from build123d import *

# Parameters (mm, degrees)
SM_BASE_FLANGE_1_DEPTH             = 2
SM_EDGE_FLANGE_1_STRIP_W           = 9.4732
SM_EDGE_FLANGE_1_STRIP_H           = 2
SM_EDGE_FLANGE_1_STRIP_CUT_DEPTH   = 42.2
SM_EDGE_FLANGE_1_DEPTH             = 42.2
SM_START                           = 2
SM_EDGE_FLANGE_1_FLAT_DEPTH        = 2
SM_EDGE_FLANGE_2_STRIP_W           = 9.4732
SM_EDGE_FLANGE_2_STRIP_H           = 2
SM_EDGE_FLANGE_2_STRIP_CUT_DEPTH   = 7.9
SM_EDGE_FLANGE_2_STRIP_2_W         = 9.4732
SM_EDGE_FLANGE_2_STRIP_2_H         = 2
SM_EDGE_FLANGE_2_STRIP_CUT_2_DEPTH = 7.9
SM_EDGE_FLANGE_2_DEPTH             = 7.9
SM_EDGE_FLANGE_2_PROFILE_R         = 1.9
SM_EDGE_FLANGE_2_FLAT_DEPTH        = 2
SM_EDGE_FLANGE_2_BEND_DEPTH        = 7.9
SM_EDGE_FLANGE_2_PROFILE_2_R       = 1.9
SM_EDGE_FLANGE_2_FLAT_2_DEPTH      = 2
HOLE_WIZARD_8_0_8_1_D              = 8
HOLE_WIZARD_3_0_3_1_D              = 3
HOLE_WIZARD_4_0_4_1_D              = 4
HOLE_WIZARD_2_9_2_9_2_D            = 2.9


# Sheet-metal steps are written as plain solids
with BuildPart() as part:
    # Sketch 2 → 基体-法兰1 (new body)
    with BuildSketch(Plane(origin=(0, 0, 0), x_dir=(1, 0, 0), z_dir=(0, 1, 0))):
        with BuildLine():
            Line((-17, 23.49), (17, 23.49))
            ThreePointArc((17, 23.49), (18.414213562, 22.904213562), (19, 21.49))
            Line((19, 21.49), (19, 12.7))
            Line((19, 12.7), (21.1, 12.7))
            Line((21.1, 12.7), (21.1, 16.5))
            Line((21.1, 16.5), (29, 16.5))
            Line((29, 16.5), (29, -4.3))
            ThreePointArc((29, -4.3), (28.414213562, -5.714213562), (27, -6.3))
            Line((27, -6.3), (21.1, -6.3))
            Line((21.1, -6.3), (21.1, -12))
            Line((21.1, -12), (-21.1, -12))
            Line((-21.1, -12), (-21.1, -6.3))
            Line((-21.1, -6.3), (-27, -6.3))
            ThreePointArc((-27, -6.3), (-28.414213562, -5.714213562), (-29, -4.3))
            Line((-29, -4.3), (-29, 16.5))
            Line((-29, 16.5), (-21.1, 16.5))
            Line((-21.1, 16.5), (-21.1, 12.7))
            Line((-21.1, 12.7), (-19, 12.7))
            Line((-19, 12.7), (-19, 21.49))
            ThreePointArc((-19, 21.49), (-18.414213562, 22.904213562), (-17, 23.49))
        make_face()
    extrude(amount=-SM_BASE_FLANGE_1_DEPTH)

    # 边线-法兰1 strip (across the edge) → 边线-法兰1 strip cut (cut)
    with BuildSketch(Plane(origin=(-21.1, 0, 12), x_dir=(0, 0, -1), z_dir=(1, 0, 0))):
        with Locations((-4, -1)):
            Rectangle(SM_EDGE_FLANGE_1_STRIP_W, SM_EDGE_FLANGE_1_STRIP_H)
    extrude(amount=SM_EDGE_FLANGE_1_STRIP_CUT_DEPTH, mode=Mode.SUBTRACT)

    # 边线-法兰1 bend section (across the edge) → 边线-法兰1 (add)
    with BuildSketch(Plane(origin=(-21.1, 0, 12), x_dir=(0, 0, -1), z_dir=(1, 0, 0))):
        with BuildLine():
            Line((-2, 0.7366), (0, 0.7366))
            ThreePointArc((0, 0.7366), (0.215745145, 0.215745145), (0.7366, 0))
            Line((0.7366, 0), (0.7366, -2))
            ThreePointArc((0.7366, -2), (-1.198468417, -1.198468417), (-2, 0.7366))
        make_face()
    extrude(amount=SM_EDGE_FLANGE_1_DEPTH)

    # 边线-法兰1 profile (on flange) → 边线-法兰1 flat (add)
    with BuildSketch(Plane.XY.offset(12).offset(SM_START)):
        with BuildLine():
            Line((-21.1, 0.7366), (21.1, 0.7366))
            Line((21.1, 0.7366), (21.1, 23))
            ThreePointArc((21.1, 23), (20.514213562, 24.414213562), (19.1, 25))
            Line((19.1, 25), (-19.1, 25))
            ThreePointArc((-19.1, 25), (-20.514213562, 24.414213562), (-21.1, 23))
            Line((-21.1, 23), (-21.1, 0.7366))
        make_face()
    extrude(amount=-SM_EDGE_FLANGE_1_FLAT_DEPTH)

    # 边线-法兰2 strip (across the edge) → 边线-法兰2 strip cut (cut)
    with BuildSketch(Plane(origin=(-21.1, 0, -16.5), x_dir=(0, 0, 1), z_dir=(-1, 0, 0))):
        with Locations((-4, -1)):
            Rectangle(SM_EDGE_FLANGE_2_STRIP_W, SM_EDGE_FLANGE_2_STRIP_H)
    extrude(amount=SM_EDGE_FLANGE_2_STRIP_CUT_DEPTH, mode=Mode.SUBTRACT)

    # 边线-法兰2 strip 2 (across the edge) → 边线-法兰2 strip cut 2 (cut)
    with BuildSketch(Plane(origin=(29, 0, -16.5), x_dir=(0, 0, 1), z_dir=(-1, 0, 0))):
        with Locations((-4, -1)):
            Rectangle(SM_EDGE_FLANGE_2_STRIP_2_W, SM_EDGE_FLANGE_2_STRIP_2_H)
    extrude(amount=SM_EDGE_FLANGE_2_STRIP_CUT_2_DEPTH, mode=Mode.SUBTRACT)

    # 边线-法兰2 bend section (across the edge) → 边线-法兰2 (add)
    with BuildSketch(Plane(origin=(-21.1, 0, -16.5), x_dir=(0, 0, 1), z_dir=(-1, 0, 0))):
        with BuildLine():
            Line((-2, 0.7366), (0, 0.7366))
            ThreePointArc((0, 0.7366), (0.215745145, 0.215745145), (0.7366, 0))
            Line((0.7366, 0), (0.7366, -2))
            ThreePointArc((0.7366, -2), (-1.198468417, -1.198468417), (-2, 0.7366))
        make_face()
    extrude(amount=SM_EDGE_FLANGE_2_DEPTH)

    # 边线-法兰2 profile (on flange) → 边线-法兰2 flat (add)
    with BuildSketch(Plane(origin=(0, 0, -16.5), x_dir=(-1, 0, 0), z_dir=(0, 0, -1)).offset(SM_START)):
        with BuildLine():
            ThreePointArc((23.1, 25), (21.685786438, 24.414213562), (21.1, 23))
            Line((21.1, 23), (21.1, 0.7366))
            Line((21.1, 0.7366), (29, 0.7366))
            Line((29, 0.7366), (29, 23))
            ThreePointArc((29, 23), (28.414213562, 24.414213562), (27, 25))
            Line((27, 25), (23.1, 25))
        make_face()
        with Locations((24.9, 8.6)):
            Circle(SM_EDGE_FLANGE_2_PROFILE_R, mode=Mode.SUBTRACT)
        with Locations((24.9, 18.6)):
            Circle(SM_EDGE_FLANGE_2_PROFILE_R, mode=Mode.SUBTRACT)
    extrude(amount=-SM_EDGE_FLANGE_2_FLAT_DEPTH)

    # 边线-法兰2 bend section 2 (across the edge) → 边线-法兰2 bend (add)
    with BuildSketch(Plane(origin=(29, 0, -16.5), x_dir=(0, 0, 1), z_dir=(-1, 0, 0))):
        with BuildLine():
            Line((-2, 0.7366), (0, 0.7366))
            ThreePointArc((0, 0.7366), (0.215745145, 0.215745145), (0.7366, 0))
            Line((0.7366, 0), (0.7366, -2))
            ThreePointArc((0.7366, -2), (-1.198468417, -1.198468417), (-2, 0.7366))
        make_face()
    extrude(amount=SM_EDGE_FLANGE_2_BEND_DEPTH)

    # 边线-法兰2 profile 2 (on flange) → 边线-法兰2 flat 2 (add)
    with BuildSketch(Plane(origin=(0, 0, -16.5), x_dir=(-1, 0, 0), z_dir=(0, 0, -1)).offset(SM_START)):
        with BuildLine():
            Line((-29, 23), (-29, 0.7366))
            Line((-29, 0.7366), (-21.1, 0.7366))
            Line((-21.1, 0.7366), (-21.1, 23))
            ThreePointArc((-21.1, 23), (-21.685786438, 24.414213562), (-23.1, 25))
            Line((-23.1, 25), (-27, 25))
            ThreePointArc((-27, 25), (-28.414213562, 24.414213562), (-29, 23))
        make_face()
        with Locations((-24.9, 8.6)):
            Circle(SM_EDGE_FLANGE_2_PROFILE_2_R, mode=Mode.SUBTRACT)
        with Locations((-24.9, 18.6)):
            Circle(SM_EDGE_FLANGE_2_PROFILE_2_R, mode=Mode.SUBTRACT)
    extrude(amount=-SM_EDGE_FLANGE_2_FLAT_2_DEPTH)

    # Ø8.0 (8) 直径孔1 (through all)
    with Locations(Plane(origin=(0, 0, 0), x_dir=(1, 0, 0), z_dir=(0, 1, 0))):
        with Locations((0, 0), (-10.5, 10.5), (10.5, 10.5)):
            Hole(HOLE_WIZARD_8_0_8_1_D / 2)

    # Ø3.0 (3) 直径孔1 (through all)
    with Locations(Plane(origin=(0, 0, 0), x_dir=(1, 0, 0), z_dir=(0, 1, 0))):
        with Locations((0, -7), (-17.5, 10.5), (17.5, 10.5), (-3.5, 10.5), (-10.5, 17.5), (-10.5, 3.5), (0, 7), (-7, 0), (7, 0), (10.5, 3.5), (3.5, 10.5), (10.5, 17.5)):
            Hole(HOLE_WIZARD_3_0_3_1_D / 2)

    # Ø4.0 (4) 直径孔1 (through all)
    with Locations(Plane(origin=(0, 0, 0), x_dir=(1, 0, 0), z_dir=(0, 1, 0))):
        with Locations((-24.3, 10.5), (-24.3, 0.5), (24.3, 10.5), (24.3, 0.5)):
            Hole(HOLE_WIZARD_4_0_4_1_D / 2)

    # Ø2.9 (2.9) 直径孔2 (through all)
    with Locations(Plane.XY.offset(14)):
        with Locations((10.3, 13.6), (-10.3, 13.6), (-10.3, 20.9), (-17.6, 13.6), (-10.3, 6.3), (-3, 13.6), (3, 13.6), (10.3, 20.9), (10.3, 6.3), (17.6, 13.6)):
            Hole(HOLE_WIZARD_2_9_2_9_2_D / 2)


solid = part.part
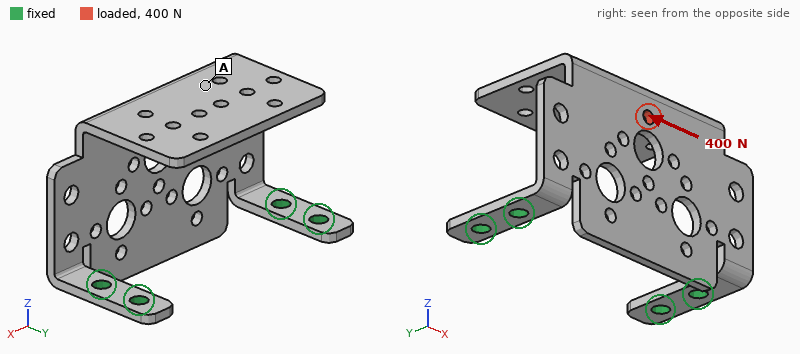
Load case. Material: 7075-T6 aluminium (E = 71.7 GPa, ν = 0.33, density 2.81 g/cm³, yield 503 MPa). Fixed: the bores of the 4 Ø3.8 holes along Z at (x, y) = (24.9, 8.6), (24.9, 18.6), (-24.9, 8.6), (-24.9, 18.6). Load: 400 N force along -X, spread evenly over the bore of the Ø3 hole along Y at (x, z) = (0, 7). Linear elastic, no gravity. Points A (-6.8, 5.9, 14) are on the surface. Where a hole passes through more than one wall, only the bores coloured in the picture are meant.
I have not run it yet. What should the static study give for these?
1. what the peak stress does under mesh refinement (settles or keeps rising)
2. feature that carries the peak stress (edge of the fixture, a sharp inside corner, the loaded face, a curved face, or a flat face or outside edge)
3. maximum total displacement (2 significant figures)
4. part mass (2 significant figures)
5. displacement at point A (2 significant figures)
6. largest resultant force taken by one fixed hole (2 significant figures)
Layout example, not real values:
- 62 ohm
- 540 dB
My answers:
- keeps rising
- edge of the fixture
- 0.27 mm
- 16 g
- 0.16 mm
- 300 N
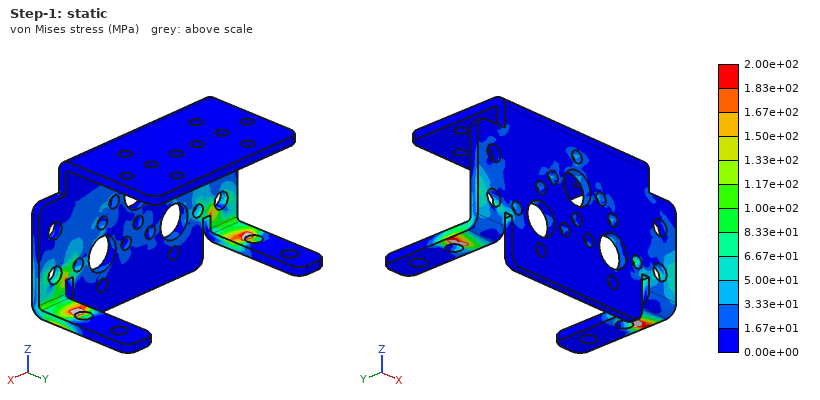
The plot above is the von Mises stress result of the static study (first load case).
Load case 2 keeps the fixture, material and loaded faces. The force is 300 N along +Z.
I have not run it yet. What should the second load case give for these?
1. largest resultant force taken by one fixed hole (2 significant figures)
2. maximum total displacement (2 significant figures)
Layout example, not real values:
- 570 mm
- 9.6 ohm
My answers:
- 150 N
- 0.49 mm
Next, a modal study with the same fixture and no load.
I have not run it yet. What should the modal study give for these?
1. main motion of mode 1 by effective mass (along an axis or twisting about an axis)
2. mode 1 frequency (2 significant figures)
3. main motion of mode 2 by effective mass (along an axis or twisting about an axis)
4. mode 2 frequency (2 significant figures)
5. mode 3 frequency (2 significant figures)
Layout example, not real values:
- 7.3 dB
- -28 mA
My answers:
- along Y
- 350 Hz
- along X
- 1100 Hz
- 1400 Hz
